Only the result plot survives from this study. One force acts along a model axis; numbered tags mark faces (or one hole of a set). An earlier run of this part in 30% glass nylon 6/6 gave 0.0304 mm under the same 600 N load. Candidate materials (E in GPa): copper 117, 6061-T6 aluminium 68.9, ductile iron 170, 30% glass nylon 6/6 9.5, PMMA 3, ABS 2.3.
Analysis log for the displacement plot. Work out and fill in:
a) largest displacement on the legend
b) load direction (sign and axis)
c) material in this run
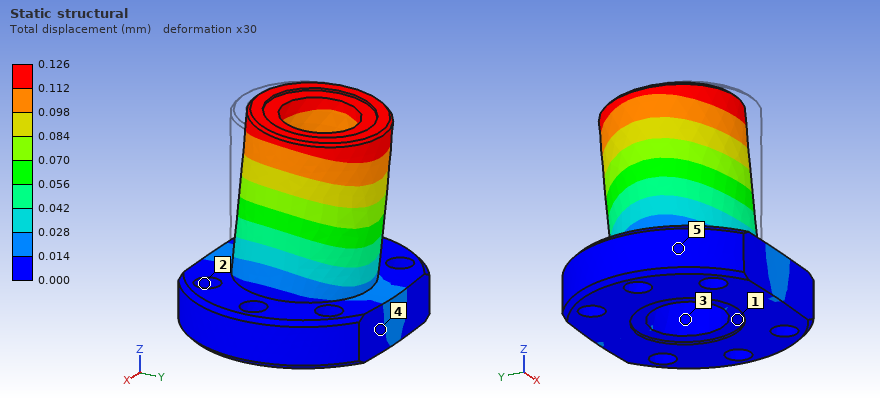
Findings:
0.126 mm
+Y
ABS
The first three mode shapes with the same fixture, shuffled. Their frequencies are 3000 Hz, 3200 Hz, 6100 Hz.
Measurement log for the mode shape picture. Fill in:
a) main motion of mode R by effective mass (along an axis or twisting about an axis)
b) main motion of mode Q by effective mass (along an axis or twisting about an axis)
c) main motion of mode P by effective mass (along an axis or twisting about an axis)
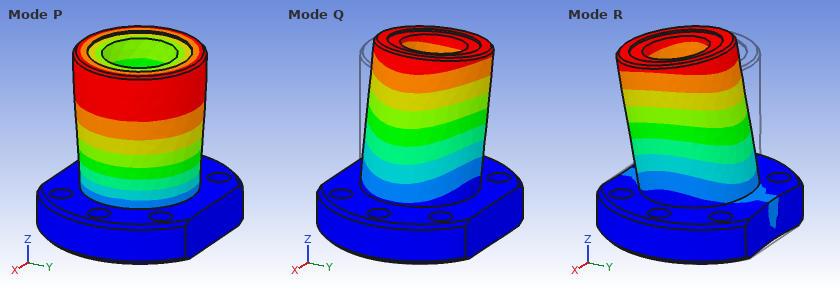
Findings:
along Y
along X
twisting about Z
